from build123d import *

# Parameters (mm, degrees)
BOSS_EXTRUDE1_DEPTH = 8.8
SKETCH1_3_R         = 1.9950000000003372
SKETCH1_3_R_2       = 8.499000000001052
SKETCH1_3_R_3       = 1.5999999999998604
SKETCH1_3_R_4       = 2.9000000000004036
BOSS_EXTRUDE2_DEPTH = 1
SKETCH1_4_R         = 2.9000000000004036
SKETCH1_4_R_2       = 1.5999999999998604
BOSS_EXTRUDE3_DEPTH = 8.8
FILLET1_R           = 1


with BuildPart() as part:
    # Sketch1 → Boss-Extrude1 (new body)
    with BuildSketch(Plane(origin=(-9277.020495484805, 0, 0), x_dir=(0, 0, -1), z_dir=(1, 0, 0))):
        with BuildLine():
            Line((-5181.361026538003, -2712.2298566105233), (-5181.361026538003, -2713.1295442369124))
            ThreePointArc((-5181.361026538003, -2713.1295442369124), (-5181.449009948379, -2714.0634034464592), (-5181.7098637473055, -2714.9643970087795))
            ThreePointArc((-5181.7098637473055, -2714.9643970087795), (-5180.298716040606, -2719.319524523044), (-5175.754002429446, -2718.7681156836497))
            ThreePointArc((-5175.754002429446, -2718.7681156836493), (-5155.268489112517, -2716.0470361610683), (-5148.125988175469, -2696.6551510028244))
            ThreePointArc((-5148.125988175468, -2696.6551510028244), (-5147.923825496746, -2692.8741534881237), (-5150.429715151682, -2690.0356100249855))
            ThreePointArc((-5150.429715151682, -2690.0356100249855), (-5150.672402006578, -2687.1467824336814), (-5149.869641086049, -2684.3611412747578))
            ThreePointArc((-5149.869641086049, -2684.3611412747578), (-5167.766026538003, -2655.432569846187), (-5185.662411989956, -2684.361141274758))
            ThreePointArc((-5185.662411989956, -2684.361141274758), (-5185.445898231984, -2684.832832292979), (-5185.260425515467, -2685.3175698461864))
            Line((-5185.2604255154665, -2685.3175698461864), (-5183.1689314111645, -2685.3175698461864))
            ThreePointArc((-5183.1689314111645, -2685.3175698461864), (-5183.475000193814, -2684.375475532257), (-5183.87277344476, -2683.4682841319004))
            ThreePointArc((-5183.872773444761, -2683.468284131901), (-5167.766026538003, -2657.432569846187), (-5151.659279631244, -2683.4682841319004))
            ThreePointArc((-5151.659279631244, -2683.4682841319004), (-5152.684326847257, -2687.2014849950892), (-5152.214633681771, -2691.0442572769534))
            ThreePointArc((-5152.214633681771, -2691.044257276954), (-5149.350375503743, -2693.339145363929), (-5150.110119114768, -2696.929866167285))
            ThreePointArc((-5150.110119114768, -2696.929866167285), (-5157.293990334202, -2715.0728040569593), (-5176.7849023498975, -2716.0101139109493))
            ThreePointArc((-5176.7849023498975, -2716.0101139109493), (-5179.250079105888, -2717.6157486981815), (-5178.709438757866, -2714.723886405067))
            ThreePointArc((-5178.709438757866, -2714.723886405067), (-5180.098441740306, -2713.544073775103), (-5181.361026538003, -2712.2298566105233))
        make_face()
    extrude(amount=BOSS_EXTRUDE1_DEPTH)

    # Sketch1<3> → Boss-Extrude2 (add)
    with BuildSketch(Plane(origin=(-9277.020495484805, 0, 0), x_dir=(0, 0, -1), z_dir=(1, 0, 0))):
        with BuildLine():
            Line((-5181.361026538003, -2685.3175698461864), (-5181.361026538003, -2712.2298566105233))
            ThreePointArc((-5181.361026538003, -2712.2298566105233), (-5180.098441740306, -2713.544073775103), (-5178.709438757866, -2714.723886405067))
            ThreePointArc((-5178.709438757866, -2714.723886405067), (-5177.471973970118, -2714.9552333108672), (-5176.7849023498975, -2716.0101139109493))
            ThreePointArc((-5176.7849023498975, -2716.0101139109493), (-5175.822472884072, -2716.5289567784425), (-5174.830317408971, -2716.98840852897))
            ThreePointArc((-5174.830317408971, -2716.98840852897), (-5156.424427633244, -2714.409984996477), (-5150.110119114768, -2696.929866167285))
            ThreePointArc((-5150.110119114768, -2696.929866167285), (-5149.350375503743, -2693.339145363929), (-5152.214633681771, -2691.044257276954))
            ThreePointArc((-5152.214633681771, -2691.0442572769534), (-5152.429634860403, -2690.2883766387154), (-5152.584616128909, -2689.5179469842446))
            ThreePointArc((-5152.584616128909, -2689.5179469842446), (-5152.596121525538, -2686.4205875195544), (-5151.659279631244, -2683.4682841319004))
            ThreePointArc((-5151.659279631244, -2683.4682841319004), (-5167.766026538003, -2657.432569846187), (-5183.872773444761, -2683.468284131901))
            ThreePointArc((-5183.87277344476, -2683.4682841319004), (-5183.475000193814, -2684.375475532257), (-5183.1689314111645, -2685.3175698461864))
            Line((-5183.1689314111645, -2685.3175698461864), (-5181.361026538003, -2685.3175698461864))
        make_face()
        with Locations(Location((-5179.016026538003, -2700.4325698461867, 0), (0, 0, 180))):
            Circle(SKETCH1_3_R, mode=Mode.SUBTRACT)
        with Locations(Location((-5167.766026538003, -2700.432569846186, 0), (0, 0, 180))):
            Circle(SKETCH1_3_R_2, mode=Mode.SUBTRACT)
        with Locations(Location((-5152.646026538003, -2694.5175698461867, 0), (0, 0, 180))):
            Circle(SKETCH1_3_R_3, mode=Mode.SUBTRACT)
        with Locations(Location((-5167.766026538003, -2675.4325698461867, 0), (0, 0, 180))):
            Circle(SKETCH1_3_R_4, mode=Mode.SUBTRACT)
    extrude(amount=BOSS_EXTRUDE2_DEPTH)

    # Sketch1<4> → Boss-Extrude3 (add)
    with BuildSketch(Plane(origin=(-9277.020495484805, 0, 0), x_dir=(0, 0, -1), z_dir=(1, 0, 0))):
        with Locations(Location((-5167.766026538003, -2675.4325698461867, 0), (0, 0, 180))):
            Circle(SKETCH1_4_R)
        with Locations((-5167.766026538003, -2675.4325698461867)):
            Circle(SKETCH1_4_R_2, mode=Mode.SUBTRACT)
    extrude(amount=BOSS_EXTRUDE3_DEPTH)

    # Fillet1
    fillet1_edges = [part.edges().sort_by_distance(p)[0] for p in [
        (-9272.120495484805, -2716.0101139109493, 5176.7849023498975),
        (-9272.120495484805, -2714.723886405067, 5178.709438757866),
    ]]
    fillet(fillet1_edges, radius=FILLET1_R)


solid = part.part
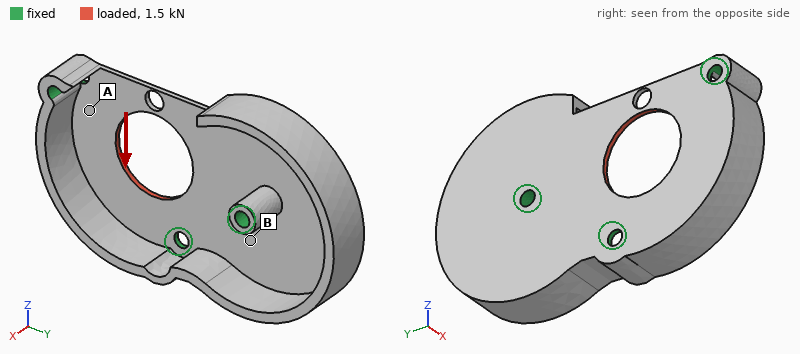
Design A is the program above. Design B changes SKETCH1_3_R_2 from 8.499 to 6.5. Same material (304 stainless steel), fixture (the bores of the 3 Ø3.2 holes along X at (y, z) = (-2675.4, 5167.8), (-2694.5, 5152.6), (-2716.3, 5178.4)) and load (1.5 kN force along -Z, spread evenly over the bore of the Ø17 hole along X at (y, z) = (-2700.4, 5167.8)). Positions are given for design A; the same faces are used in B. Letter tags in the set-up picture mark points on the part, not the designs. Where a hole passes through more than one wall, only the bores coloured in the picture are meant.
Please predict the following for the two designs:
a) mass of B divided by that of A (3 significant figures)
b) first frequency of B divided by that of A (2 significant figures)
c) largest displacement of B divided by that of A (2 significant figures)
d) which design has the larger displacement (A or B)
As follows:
1.02
1.0
0.70
A
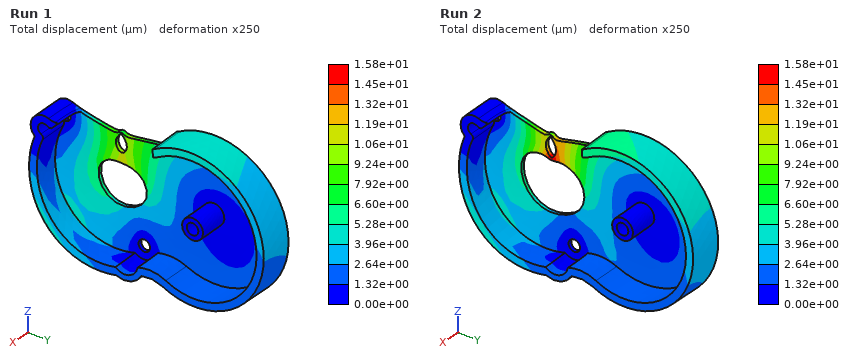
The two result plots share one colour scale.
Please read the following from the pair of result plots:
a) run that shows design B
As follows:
Run 1
